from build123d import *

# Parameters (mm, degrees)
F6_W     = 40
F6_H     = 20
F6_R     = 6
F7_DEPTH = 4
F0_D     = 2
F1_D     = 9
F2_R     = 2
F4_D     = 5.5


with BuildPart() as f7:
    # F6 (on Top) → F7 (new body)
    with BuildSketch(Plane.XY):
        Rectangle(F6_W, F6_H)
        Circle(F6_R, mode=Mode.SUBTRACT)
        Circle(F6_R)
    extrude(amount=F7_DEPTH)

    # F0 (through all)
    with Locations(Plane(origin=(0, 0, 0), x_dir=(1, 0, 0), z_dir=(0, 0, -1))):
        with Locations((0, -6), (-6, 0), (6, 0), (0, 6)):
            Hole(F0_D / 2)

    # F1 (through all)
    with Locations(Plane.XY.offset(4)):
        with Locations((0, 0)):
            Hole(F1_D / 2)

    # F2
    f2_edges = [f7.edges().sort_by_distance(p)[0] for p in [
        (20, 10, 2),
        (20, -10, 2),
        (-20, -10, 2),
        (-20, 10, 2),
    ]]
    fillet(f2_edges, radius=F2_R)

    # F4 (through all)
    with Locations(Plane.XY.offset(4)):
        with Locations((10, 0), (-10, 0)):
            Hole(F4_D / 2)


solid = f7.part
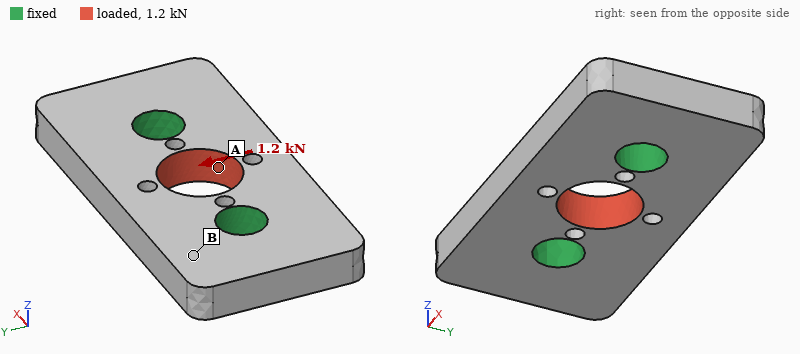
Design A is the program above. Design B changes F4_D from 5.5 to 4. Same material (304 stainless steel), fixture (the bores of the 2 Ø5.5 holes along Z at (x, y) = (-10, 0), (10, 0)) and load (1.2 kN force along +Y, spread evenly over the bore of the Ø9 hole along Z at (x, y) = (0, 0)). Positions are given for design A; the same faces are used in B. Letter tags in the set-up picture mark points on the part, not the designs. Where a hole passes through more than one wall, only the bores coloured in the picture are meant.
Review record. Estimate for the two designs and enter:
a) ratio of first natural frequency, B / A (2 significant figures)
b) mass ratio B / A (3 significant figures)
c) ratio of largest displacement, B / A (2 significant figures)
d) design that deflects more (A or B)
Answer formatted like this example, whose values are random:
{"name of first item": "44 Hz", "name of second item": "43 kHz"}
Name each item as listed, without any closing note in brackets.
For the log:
{"ratio of first natural frequency, B / A": "0.81", "mass ratio B / A": "1.03", "ratio of largest displacement, B / A": "1.1", "design that deflects more": "B"}
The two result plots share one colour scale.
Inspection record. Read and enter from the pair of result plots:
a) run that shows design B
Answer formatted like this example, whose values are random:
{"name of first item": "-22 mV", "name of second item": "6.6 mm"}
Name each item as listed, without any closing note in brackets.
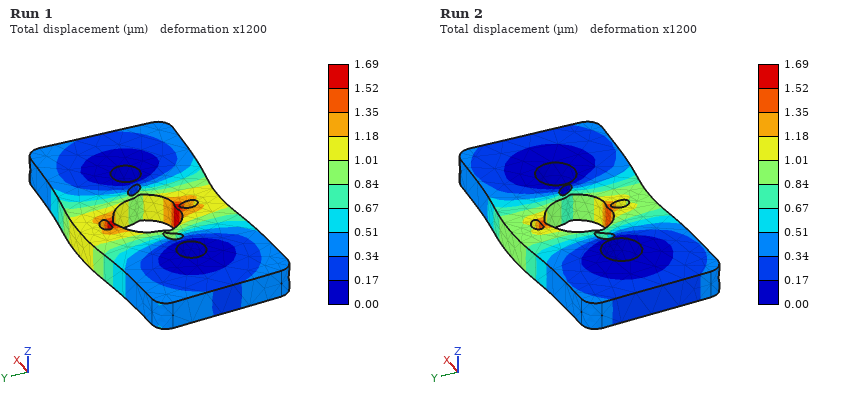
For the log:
{"run that shows design B": "Run 1"}
